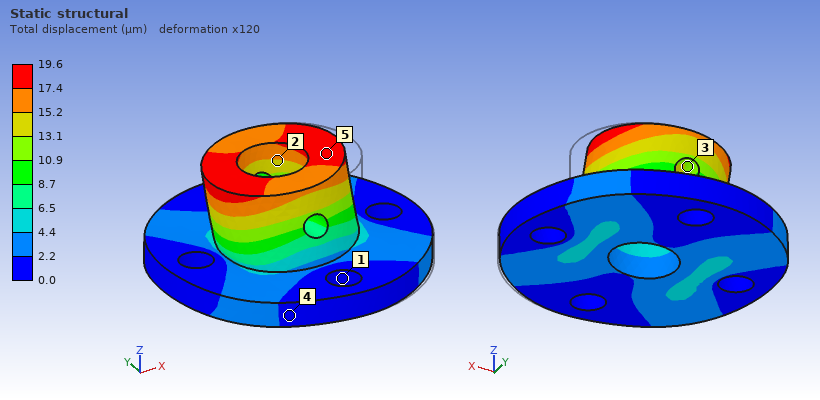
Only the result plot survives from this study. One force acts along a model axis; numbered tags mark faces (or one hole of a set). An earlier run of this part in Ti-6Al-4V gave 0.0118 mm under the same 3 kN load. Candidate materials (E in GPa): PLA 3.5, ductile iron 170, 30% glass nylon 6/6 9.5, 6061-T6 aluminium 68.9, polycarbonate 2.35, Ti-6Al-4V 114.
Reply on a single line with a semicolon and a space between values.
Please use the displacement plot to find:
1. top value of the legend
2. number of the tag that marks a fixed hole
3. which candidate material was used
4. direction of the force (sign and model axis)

19.6 µm; 1; 6061-T6 aluminium; -X
